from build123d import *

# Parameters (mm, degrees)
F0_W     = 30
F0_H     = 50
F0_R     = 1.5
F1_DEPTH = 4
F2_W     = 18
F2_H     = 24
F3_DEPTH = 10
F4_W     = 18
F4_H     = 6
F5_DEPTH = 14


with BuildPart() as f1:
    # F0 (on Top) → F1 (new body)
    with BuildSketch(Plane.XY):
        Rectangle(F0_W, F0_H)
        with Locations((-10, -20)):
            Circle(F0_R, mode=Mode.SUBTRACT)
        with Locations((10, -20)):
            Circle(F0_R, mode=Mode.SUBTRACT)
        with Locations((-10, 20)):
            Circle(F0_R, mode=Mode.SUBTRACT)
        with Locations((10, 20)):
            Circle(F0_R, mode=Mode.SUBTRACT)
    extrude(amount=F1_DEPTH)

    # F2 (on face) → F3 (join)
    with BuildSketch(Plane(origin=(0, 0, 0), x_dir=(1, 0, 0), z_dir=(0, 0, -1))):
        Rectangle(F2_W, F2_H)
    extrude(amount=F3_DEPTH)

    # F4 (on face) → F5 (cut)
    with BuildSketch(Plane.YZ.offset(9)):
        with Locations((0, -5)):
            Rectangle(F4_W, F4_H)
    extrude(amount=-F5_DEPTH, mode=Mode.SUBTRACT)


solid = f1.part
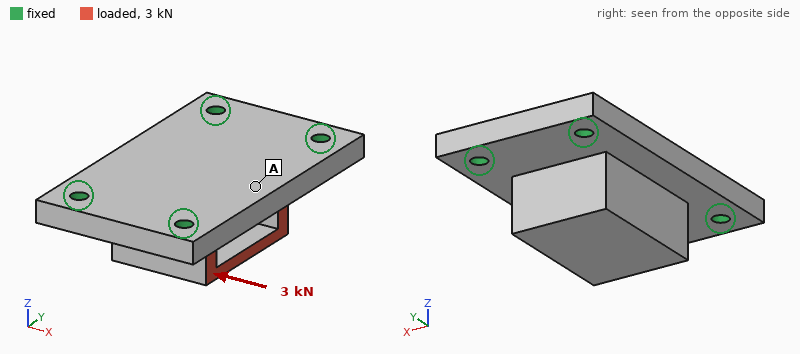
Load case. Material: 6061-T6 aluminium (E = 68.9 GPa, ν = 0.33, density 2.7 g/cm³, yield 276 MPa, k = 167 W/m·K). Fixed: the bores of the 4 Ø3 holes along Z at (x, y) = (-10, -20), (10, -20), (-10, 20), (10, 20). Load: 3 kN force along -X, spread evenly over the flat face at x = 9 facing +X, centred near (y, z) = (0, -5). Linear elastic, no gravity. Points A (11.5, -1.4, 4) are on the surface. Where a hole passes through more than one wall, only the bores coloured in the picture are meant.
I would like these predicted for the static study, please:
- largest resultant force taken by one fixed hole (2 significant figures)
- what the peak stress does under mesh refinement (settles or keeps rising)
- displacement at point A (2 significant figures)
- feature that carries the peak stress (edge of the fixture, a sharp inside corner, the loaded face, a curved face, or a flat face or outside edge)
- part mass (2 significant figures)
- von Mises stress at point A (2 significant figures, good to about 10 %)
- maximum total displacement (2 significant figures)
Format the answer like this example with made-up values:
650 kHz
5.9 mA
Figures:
1.1 kN
keeps rising
26 µm
edge of the fixture
23 g
25 MPa
43 µm
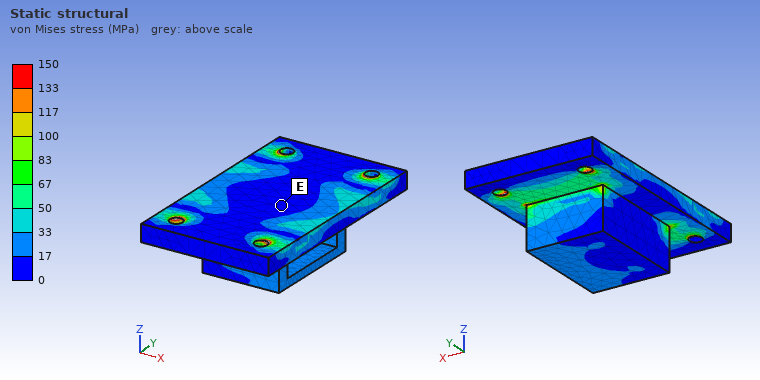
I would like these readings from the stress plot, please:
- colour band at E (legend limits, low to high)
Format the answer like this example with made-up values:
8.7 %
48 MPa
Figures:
0 to 17 MPa
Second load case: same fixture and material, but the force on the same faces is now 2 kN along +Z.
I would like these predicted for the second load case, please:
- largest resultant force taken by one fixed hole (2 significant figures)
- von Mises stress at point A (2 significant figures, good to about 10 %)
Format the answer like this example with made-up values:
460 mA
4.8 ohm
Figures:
970 N
39 MPa
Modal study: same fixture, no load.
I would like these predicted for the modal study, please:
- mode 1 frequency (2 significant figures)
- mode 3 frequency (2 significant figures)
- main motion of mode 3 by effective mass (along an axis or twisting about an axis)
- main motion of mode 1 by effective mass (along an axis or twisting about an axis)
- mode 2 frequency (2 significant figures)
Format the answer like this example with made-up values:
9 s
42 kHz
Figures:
12 kHz
20 kHz
along Y
along Z
14 kHz
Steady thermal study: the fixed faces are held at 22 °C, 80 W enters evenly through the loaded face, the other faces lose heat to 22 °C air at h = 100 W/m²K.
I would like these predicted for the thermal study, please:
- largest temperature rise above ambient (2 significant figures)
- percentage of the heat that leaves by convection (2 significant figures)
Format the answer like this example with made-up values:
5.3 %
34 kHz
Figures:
64 K
12 %
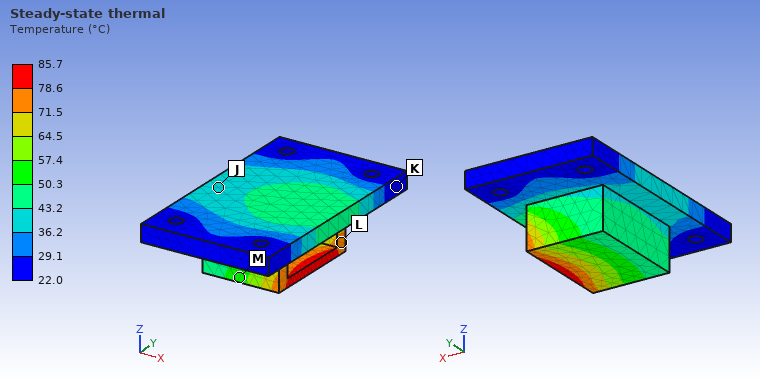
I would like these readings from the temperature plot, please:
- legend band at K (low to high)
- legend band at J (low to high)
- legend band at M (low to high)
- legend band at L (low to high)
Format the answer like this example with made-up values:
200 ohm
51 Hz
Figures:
22.0 to 29.1 °C
36.2 to 43.2 °C
50.3 to 57.4 °C
71.5 to 78.6 °C
